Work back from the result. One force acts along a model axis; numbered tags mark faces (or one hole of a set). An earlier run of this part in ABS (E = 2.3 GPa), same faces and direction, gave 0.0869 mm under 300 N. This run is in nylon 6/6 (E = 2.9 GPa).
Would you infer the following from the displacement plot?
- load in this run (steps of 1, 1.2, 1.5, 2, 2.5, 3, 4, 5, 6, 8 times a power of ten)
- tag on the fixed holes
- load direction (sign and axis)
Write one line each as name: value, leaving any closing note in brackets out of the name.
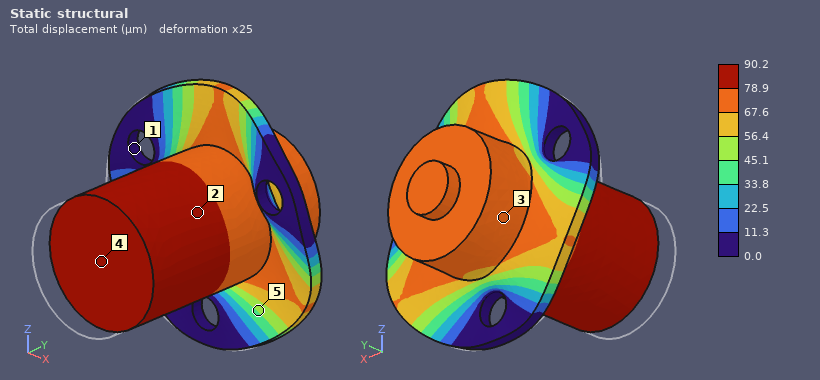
load in this run: 400 N
tag on the fixed holes: 1
load direction: +Y
